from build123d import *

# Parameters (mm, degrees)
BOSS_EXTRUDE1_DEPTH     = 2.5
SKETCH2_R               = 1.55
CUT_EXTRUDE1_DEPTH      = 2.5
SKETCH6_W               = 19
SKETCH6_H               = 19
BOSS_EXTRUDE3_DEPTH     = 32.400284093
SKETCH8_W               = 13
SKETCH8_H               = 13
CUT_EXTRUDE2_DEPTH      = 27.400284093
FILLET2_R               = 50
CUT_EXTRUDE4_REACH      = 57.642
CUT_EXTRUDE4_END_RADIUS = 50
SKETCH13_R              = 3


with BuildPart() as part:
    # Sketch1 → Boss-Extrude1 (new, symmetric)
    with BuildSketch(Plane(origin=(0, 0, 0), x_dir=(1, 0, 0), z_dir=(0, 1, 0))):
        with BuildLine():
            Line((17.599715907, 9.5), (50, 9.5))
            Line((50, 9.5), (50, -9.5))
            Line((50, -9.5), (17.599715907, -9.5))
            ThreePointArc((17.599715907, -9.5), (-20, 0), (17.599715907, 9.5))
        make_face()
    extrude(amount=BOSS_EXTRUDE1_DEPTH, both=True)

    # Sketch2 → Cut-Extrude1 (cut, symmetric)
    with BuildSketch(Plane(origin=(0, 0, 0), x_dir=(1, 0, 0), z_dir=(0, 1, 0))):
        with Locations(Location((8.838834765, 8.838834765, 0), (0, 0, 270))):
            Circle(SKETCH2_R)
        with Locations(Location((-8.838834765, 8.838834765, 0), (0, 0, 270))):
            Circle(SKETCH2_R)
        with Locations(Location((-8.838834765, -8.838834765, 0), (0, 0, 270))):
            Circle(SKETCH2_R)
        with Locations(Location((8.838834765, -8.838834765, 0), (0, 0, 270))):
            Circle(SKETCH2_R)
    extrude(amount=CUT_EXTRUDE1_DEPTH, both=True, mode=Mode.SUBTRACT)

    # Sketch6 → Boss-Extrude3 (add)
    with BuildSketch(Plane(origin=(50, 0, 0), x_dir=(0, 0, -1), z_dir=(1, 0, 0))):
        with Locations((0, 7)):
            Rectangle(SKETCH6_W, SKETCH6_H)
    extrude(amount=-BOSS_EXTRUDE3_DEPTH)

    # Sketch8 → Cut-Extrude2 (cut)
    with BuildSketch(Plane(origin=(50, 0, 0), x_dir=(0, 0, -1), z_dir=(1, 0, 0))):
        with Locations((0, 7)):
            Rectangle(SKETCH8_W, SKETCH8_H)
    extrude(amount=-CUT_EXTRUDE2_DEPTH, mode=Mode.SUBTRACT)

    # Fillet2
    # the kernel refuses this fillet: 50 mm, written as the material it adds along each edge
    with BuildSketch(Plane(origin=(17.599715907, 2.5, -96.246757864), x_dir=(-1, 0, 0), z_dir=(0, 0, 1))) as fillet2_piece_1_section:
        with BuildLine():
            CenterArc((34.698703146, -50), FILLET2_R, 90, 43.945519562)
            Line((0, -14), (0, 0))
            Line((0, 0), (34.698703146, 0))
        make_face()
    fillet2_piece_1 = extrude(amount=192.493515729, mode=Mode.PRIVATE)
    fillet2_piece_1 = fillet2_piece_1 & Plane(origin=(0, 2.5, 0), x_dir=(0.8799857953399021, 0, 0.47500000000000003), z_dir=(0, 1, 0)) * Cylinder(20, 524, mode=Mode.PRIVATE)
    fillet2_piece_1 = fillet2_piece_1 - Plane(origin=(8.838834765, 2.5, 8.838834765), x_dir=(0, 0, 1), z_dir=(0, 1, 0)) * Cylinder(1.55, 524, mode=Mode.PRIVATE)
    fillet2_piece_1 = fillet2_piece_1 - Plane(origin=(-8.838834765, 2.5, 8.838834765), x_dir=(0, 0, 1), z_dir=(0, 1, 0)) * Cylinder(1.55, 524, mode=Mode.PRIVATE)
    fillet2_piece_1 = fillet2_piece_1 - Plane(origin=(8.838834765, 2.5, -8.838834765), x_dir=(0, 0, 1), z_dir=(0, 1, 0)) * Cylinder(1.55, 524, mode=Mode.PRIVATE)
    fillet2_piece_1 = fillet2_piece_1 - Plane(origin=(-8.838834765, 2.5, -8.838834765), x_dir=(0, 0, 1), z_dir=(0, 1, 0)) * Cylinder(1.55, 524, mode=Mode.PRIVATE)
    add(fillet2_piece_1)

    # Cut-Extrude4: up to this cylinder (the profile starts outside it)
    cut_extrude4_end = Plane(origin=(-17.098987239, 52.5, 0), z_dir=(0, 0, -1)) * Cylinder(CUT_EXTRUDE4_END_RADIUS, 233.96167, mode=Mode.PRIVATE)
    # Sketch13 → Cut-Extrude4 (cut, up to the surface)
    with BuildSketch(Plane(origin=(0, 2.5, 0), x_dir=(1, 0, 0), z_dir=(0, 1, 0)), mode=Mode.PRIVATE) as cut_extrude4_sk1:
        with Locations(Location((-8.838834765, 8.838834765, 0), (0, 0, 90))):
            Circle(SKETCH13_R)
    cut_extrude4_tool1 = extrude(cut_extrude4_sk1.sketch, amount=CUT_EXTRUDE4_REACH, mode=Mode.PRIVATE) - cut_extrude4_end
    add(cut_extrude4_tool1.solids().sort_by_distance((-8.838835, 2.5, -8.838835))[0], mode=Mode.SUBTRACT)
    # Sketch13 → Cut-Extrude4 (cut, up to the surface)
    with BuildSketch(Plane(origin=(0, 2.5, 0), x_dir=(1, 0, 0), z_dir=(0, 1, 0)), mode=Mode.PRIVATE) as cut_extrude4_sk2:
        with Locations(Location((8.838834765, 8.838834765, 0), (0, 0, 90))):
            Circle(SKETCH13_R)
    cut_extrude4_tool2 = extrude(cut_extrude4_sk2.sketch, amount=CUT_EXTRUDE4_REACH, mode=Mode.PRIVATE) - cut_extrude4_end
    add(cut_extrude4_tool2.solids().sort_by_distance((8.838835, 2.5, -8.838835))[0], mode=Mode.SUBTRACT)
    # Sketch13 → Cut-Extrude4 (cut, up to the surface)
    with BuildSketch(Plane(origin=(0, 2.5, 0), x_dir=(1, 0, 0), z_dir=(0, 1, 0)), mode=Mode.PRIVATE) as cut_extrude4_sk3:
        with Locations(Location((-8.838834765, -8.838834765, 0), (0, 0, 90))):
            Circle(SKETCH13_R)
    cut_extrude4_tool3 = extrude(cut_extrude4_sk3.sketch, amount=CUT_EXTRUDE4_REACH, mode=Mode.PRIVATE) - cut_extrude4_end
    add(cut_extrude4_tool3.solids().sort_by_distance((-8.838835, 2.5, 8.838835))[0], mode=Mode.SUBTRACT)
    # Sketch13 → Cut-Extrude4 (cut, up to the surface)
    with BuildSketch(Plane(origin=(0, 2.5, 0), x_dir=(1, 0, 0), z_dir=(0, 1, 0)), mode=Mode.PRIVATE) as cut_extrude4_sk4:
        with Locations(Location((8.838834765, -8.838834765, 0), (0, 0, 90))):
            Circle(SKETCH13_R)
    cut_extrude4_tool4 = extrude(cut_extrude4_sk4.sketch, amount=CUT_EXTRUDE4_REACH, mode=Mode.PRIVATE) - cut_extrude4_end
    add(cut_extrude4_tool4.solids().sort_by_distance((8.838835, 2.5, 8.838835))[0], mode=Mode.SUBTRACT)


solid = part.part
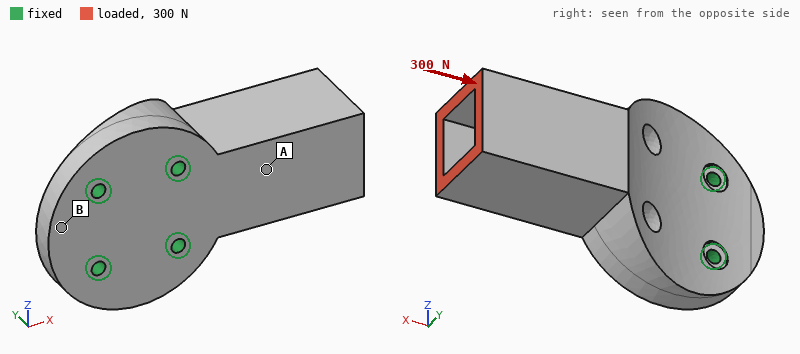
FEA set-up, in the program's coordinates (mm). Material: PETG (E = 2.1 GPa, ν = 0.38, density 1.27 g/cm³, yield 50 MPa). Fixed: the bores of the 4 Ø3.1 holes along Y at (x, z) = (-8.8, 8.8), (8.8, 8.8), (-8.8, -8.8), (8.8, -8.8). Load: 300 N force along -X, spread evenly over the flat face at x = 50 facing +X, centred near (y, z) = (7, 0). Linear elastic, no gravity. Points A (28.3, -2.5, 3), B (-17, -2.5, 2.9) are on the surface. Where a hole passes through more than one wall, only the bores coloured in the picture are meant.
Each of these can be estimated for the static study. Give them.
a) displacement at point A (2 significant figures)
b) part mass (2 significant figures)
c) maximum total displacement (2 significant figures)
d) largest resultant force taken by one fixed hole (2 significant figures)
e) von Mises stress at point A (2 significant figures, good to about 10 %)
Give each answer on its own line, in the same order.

0.060 mm
22 g
0.16 mm
97 N
1.5 MPa
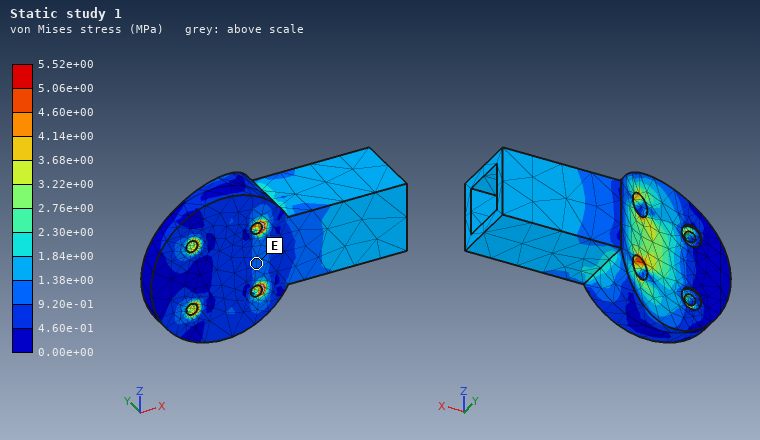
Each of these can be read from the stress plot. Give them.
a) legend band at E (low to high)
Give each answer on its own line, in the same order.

9.20e-01 to 1.38e+00 MPa
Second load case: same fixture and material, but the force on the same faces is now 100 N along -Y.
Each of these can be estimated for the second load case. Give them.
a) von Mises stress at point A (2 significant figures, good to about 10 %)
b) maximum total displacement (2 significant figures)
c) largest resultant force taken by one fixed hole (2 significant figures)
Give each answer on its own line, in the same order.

2.5 MPa
0.49 mm
170 N
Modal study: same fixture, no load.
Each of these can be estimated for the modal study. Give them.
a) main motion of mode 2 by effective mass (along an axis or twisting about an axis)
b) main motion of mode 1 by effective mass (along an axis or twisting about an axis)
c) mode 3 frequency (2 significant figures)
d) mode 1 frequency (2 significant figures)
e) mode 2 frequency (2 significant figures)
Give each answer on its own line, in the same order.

along Z
along Y
4000 Hz
1300 Hz
2200 Hz
